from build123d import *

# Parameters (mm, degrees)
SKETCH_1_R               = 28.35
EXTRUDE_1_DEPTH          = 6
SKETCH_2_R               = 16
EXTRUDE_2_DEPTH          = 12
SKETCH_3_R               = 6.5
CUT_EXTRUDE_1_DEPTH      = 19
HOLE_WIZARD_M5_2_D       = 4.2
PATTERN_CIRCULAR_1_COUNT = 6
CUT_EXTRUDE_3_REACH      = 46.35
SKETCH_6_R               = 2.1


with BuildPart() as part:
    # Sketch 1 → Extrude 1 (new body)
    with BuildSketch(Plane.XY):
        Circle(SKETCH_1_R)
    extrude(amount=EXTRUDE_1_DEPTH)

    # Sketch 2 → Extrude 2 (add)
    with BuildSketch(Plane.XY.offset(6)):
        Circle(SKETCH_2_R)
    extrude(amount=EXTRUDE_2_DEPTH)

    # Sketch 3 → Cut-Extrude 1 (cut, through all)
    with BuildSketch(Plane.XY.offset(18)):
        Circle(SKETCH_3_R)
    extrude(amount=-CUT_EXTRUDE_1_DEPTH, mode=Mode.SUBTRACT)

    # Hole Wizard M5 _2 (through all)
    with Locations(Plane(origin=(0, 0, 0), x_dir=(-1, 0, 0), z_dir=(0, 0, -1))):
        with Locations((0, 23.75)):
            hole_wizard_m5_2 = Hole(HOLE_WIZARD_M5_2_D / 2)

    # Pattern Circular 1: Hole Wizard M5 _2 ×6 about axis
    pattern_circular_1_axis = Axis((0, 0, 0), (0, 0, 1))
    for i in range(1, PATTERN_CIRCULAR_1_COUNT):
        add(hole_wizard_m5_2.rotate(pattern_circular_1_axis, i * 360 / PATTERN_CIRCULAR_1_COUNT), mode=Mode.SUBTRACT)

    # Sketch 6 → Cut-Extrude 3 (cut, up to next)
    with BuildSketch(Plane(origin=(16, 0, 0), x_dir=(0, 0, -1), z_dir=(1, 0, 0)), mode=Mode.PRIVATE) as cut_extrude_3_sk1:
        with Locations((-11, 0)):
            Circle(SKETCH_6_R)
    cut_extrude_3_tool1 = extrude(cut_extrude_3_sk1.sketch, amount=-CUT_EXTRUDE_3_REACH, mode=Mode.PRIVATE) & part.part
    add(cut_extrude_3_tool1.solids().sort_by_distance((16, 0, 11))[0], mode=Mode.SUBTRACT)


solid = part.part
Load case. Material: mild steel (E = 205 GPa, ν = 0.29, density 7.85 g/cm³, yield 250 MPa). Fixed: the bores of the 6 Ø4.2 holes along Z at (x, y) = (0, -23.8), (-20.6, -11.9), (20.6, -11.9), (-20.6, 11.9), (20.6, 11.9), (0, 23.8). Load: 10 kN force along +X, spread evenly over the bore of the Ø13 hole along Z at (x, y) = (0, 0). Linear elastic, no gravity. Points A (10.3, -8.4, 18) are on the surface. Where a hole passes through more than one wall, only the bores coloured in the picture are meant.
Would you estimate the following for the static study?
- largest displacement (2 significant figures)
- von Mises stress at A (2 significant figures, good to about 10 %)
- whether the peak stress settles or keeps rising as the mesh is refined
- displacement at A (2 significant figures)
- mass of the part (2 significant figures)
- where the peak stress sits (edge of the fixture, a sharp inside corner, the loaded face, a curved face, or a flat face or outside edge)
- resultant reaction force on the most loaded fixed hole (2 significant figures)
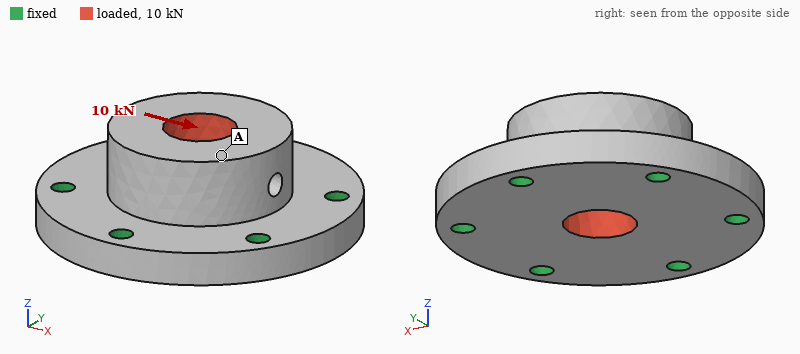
5.4 µm
11 MPa
keeps rising
4.7 µm
170 g
edge of the fixture
2.3 kN
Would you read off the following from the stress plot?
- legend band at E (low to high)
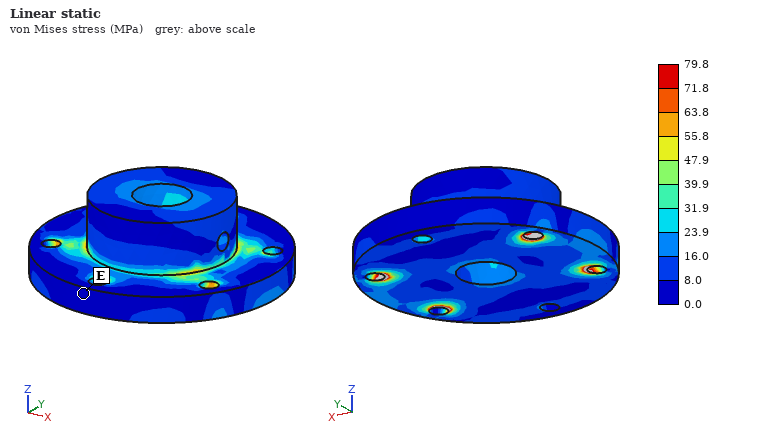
0.0 to 8.0 MPa
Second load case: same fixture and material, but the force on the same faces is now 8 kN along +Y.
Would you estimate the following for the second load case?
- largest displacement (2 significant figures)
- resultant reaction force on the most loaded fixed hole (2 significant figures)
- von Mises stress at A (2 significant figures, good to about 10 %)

4.3 µm
2.1 kN
6.9 MPa
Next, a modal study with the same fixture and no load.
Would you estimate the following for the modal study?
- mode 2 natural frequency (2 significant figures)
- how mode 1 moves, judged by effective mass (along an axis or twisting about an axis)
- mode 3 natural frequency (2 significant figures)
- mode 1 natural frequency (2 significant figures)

24 kHz
along Z
24 kHz
21 kHz
